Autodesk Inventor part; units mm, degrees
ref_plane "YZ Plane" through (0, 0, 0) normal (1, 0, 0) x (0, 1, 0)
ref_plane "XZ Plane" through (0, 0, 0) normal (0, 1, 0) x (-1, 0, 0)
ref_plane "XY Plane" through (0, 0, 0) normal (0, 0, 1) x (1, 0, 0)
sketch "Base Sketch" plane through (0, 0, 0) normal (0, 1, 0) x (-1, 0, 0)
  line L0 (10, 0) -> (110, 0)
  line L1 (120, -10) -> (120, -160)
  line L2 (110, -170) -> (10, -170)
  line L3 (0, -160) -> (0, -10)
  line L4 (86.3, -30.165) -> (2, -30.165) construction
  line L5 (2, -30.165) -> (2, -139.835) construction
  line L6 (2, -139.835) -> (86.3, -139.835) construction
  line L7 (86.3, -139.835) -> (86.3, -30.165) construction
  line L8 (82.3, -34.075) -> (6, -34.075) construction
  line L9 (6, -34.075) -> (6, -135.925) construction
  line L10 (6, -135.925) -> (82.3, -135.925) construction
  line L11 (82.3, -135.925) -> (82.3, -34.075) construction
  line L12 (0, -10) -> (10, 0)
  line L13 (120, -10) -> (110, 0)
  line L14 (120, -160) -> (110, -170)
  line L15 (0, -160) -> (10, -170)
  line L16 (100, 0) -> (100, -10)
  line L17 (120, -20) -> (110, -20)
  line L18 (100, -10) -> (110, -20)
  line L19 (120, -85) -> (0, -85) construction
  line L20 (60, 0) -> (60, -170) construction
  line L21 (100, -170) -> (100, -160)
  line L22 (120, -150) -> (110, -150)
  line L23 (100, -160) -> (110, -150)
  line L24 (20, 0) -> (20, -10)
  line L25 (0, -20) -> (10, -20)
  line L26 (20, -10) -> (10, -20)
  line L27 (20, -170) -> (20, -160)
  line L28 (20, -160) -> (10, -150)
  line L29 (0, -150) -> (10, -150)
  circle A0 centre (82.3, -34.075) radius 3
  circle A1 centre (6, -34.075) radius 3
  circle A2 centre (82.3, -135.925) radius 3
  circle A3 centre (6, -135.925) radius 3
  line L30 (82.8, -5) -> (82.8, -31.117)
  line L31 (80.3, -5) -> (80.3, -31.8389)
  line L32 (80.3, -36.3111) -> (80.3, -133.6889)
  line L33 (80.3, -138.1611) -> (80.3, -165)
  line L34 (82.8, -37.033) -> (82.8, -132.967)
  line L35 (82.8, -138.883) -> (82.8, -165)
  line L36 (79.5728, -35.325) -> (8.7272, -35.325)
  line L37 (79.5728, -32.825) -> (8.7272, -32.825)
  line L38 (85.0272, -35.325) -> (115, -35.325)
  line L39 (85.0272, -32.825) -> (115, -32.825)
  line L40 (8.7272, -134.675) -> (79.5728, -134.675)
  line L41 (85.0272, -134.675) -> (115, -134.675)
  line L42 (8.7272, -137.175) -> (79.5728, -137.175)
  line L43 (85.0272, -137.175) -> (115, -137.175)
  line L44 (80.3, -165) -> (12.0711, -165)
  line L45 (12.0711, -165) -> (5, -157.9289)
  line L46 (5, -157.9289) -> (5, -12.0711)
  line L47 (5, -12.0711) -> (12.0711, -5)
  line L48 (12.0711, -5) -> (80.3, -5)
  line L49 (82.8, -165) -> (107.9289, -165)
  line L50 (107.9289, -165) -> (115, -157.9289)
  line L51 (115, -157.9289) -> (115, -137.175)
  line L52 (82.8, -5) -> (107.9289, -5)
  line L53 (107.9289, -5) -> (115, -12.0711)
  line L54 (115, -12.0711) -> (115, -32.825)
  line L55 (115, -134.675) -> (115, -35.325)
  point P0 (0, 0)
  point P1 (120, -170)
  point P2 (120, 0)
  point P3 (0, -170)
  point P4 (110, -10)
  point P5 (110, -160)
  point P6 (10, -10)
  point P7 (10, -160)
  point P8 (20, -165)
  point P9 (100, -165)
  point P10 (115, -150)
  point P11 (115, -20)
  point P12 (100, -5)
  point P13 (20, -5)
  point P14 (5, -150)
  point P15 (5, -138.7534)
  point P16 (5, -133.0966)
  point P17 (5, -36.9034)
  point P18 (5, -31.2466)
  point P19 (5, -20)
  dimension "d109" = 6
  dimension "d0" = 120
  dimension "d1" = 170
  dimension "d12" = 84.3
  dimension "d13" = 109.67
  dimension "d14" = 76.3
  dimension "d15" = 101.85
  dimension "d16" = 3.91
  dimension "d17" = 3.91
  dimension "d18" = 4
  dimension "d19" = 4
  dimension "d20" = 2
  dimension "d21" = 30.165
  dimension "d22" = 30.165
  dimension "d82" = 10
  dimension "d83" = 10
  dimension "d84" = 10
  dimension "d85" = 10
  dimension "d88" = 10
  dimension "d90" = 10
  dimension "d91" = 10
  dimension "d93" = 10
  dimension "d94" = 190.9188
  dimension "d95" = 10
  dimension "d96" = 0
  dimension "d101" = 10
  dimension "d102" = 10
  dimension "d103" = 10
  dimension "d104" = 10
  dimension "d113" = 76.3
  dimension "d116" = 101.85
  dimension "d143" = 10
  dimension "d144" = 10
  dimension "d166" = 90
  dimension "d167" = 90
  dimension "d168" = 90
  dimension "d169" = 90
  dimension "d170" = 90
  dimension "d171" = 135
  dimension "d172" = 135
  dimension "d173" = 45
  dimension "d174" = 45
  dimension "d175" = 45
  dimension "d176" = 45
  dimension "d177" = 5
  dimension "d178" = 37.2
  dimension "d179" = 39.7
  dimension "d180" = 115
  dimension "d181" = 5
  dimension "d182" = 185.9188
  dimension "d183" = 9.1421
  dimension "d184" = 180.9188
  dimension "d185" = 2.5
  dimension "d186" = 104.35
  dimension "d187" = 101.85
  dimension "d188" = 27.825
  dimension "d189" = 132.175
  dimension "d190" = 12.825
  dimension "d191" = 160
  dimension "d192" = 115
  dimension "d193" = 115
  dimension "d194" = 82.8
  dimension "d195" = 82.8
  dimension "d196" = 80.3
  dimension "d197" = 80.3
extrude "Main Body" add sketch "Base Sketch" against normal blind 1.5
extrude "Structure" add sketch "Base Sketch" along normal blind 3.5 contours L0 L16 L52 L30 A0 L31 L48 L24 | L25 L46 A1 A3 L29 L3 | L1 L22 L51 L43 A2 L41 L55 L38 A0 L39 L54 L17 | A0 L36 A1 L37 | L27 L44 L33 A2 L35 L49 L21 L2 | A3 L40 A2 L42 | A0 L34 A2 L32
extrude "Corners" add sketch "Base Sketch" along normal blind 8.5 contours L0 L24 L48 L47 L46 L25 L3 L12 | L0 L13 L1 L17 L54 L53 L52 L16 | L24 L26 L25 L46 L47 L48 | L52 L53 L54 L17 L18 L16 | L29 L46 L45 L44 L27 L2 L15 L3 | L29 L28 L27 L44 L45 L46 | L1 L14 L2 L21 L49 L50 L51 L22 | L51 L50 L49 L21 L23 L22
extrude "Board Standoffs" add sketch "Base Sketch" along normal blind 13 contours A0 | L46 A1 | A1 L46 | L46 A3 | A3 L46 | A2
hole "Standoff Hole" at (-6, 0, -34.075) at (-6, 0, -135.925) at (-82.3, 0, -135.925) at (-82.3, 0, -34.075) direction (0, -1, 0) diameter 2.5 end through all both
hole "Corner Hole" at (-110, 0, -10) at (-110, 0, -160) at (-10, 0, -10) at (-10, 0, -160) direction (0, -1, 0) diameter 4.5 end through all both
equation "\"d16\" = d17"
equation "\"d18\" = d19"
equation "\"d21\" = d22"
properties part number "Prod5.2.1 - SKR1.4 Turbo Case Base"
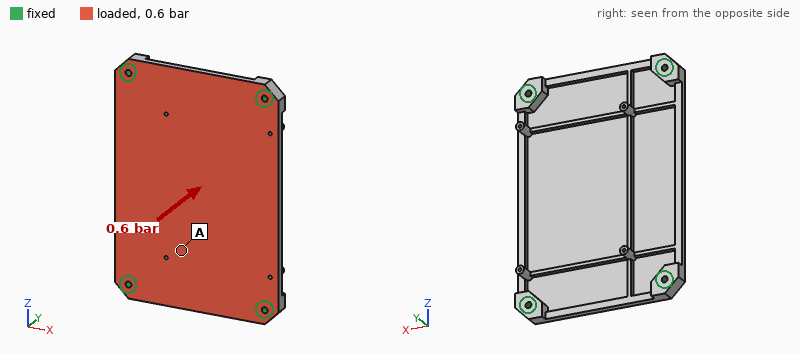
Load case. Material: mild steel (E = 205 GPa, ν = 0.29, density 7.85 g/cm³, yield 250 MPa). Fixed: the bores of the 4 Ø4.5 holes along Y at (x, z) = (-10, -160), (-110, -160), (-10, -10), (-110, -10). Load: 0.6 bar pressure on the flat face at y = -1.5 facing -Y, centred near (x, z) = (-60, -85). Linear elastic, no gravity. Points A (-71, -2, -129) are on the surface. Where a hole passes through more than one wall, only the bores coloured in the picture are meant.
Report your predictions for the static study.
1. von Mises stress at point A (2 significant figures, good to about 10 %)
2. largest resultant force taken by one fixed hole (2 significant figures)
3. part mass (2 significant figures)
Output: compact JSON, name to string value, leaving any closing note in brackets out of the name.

{"von Mises stress at point A": "26 MPa", "largest resultant force taken by one fixed hole": "370 N", "part mass": "400 g"}
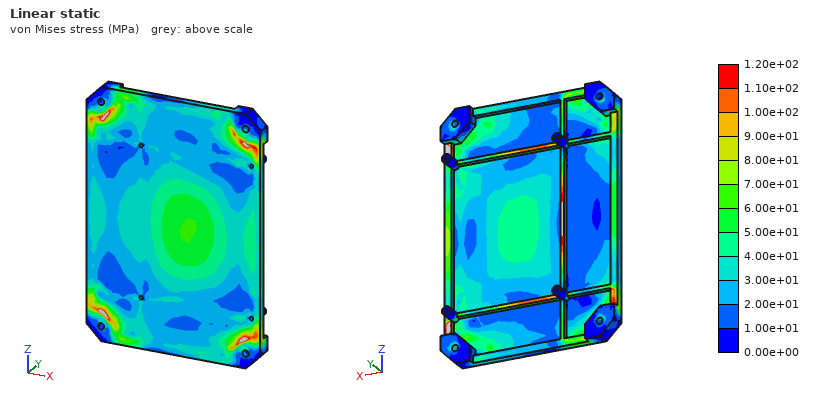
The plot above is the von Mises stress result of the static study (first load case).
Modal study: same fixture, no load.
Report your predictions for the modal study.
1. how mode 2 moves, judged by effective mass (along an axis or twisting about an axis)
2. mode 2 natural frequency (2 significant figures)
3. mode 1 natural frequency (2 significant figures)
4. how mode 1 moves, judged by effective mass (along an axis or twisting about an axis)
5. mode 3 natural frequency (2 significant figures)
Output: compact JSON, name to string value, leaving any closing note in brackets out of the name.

{"how mode 2 moves, judged by effective mass": "twisting about Z", "mode 2 natural frequency": "1200 Hz", "mode 1 natural frequency": "700 Hz", "how mode 1 moves, judged by effective mass": "along Y", "mode 3 natural frequency": "1400 Hz"}
